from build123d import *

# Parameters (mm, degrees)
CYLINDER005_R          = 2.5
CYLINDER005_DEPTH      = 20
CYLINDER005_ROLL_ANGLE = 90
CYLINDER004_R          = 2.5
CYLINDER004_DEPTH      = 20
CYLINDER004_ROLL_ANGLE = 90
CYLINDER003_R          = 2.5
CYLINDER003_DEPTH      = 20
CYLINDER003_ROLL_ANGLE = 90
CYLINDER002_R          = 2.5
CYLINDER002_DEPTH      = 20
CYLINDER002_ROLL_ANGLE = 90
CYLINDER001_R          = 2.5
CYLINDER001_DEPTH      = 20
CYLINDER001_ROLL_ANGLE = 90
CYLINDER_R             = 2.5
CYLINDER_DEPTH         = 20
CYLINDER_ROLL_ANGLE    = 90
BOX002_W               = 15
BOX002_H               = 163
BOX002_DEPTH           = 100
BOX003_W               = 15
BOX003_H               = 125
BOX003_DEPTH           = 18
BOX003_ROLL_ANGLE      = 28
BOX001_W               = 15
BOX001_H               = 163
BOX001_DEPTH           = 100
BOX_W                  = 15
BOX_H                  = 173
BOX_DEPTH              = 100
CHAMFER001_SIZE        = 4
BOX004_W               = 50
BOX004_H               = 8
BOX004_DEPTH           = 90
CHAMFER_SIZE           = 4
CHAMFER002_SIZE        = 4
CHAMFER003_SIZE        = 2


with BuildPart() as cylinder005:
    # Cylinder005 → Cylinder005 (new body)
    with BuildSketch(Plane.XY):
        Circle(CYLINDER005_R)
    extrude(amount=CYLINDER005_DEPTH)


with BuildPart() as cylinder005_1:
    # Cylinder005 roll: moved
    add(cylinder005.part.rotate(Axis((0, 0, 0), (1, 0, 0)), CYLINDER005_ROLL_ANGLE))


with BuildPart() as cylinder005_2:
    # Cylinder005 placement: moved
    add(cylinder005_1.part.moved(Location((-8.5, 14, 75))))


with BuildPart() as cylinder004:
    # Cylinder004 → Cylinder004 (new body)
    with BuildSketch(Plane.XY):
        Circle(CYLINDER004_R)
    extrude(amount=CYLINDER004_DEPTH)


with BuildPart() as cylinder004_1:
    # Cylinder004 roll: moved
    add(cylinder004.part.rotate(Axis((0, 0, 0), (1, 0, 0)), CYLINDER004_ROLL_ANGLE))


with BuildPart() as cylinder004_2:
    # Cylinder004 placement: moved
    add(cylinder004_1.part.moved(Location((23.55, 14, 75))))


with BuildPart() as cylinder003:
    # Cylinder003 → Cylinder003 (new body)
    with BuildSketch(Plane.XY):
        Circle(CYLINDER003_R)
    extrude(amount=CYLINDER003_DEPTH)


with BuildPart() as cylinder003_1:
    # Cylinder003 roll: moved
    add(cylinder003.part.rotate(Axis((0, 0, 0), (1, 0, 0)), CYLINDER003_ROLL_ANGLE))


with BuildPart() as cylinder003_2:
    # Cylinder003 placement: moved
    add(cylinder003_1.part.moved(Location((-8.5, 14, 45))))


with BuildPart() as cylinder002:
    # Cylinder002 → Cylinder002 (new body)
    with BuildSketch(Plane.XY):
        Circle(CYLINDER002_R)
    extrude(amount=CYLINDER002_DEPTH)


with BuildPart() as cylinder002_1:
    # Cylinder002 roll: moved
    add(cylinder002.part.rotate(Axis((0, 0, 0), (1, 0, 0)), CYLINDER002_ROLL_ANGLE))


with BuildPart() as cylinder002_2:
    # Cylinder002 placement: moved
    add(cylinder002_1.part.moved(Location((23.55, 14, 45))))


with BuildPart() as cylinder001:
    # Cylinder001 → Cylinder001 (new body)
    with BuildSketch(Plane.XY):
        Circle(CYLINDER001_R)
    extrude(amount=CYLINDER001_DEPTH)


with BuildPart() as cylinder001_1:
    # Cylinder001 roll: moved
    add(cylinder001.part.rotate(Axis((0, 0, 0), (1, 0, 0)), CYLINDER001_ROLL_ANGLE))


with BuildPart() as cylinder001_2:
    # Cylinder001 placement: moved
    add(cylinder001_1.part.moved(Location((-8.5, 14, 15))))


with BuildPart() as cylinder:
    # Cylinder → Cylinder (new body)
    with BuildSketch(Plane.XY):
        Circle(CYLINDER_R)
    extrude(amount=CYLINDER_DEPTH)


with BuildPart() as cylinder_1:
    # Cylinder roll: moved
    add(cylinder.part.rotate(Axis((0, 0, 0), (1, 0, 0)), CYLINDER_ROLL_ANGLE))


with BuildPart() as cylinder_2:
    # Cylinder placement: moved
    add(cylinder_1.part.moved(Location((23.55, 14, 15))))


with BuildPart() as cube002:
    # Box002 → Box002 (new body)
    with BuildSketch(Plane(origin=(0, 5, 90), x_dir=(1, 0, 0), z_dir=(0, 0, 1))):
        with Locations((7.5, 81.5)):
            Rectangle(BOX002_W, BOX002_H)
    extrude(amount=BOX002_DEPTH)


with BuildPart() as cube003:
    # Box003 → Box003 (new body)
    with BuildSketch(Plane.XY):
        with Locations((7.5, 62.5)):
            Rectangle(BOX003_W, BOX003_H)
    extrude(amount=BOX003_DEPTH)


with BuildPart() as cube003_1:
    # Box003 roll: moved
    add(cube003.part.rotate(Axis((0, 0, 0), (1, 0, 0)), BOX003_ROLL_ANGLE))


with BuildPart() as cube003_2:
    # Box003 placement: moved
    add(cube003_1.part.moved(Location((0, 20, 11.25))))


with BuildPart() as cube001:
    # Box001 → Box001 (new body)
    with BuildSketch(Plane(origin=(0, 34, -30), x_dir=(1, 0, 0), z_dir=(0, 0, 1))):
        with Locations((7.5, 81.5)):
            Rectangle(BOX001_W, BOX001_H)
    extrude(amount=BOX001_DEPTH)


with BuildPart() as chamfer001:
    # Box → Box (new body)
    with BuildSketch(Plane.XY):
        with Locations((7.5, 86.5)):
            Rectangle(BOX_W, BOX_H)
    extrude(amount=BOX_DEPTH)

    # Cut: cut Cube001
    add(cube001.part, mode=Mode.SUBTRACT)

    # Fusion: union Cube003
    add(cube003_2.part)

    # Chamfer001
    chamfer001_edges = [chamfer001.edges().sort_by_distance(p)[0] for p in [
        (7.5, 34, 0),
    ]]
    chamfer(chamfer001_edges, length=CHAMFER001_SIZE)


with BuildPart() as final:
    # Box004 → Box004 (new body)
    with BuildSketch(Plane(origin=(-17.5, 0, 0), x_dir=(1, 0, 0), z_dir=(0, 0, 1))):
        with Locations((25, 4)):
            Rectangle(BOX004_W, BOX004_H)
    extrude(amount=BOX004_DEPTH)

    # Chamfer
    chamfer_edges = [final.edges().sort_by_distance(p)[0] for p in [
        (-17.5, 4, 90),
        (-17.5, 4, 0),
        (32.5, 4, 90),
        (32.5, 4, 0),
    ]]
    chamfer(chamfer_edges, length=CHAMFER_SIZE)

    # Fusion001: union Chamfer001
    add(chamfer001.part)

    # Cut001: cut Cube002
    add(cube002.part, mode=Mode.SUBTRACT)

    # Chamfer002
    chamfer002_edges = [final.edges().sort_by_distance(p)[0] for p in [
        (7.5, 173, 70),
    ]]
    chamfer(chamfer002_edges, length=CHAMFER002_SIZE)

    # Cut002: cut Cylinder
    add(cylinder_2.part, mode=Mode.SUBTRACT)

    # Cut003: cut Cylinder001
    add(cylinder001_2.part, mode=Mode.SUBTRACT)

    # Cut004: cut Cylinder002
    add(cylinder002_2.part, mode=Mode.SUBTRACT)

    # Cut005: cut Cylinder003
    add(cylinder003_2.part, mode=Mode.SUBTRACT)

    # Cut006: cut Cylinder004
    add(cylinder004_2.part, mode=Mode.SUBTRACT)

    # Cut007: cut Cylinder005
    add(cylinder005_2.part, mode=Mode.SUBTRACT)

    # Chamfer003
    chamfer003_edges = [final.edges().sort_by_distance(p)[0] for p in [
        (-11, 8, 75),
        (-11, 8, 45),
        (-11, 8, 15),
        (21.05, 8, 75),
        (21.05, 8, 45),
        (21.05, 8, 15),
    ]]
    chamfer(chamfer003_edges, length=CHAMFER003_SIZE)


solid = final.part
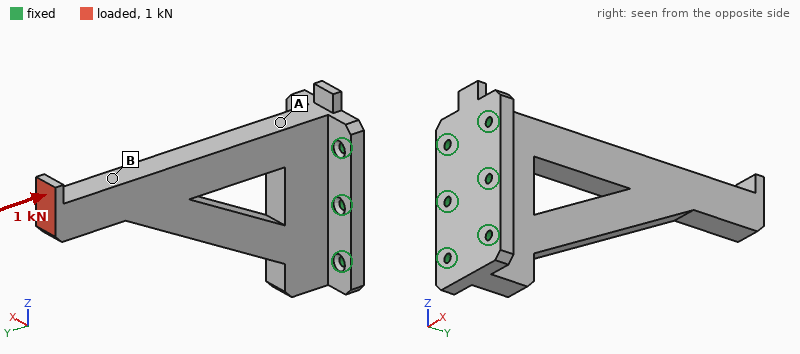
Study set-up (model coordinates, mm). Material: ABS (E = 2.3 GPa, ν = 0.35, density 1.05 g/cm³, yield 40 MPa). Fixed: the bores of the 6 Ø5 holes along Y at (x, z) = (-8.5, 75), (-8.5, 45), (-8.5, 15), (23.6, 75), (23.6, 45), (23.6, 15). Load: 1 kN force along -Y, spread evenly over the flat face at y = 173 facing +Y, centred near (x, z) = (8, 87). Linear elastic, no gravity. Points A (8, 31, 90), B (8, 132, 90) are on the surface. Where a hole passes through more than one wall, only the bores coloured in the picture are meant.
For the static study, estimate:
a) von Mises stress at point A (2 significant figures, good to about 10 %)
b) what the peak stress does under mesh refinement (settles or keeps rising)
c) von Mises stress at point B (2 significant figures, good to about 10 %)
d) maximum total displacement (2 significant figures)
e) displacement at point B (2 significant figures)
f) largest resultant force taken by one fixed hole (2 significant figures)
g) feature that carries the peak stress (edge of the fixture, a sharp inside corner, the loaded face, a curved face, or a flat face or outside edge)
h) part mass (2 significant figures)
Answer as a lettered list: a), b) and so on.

a) 3.5 MPa
b) keeps rising
c) 10 MPa
d) 2.0 mm
e) 0.80 mm
f) 560 N
g) edge of the fixture
h) 140 g
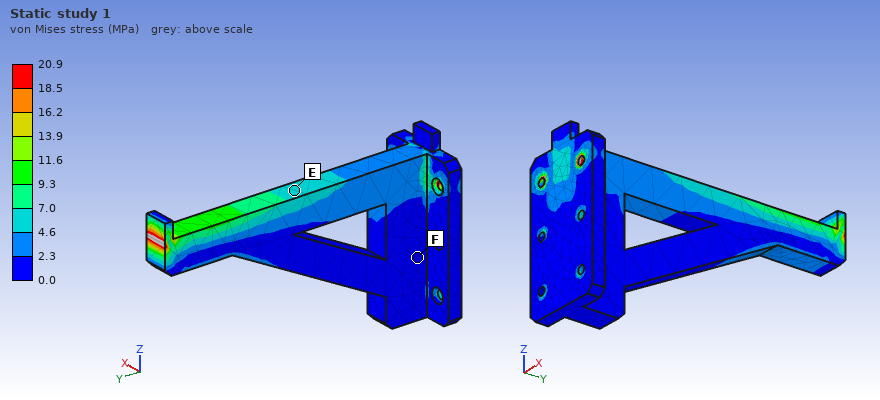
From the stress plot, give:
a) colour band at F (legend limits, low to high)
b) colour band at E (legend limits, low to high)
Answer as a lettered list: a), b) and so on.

a) 0.0 to 2.3 MPa
b) 4.6 to 7.0 MPa
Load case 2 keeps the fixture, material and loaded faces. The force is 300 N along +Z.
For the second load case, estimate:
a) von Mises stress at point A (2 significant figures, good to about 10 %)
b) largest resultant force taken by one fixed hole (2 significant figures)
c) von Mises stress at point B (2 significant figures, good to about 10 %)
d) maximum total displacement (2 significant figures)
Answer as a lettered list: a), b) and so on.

a) 3.0 MPa
b) 450 N
c) 12 MPa
d) 2.4 mm
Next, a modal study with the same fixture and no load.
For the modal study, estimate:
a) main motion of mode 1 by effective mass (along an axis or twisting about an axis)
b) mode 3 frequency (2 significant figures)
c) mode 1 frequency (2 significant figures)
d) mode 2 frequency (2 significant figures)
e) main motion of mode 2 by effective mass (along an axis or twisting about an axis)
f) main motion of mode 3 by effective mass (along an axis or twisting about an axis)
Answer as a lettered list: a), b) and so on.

a) along X
b) 790 Hz
c) 170 Hz
d) 540 Hz
e) along Z
f) along X
